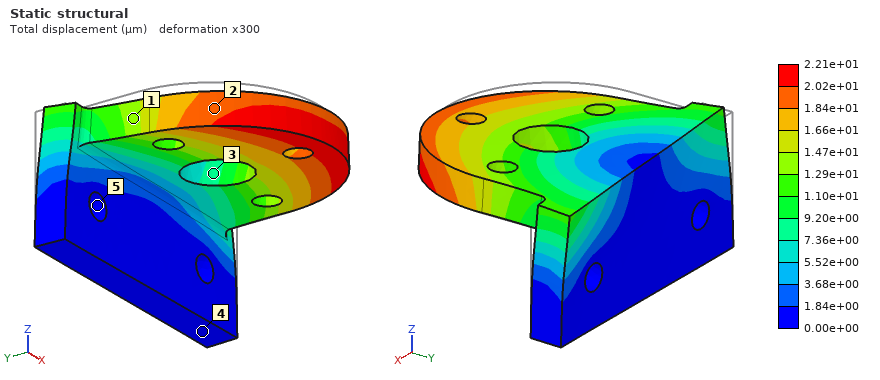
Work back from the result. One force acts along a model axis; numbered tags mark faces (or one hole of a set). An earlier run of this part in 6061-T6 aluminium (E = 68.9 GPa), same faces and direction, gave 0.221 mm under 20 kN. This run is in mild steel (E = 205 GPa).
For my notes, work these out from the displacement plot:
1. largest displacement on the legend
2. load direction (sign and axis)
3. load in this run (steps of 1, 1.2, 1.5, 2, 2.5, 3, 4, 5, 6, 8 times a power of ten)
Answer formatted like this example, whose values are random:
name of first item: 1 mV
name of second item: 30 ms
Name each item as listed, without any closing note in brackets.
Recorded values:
largest displacement on the legend: 2.21e+01 µm
load direction: +X
load in this run: 6 kN
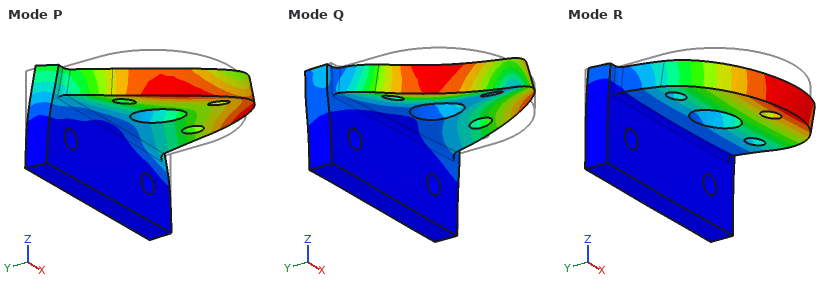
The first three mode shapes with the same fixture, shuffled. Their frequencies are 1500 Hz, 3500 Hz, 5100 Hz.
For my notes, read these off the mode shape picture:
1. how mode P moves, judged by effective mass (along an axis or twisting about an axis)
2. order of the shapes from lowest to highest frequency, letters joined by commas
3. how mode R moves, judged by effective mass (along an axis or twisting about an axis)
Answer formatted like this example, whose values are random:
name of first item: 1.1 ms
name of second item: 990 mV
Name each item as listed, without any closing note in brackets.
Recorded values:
how mode P moves, judged by effective mass: along X
order of the shapes from lowest to highest frequency, letters joined by commas: R, P, Q
how mode R moves, judged by effective mass: along Z
